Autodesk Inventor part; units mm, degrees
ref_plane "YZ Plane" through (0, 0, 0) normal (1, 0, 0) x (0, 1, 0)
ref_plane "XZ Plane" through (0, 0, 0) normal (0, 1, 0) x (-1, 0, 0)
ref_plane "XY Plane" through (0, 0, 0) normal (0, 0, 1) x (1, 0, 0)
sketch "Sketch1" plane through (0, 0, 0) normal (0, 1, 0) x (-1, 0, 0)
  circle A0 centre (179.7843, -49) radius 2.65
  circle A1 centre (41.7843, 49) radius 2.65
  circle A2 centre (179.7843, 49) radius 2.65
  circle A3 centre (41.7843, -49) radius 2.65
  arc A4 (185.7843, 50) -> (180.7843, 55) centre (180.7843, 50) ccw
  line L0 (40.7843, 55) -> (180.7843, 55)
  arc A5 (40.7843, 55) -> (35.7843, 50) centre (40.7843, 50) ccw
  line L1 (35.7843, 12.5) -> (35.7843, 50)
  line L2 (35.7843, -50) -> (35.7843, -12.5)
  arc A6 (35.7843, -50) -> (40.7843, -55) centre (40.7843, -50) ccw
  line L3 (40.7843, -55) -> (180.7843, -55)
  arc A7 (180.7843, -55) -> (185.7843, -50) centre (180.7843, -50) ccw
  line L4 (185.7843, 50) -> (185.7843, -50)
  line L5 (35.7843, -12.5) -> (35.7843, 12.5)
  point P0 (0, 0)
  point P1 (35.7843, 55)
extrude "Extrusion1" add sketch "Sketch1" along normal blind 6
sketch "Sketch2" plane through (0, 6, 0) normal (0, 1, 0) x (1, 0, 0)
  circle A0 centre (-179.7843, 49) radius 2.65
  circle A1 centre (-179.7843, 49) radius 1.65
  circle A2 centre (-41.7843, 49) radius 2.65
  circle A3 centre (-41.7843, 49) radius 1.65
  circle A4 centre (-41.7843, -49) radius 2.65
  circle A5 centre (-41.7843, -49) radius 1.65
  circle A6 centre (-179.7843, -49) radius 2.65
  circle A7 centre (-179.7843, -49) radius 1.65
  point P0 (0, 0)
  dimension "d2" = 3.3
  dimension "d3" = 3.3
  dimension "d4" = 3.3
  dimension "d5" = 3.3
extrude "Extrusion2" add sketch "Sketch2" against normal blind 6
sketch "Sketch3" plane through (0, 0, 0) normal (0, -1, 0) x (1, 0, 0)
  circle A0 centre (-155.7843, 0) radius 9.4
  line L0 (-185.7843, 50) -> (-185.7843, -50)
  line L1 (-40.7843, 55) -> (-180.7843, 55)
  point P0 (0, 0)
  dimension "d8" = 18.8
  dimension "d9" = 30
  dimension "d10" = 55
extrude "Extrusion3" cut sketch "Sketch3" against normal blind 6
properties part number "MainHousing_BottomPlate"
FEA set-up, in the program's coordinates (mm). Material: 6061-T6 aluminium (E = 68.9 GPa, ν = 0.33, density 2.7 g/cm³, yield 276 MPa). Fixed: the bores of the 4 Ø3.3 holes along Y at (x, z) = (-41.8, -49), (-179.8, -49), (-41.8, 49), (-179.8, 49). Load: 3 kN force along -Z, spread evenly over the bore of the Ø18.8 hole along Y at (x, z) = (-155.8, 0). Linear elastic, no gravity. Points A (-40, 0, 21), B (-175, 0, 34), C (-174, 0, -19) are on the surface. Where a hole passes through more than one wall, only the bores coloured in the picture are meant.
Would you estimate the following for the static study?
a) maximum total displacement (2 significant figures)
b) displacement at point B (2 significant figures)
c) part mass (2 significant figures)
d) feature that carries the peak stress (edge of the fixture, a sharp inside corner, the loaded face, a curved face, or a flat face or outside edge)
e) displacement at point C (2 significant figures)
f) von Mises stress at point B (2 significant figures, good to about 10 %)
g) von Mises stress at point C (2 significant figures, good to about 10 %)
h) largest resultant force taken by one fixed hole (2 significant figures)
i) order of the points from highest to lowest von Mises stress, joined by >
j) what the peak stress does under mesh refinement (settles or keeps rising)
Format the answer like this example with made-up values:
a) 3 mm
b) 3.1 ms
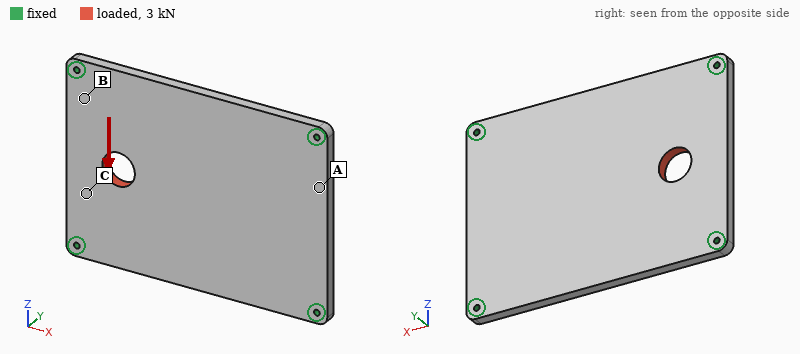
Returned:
a) 9.0 µm
b) 3.5 µm
c) 260 g
d) edge of the fixture
e) 4.9 µm
f) 9.8 MPa
g) 6.5 MPa
h) 1.2 kN
i) B > C > A
j) keeps rising
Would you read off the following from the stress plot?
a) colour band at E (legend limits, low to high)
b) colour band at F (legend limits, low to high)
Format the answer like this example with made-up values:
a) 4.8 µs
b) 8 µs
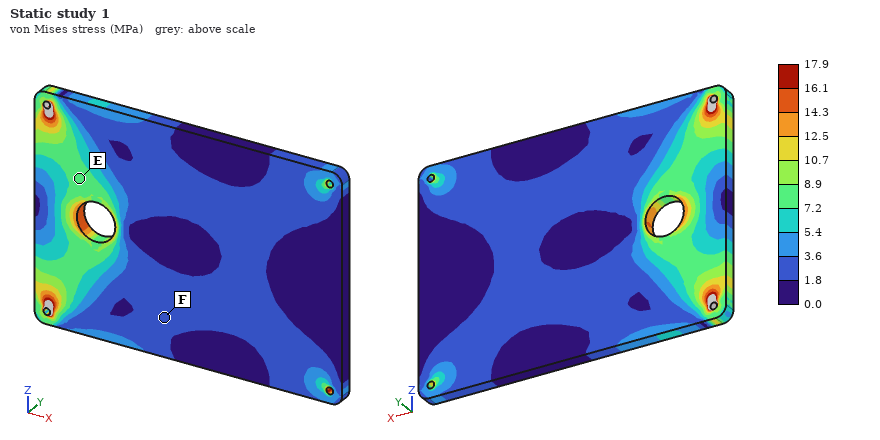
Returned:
a) 7.2 to 8.9 MPa
b) 1.8 to 3.6 MPa
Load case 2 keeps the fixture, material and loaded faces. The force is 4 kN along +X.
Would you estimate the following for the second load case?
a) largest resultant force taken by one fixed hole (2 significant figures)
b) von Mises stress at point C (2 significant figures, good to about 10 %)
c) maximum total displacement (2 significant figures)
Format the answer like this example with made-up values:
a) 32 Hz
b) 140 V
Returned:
a) 1.3 kN
b) 6.8 MPa
c) 15 µm
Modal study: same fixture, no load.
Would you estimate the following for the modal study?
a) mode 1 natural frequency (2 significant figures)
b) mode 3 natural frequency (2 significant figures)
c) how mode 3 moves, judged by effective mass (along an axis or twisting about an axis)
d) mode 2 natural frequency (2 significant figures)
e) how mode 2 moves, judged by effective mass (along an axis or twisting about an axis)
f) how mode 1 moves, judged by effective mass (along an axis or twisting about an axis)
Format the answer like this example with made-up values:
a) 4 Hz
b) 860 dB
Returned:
a) 1100 Hz
b) 2700 Hz
c) twisting about Z
d) 1900 Hz
e) twisting about X
f) along Y
